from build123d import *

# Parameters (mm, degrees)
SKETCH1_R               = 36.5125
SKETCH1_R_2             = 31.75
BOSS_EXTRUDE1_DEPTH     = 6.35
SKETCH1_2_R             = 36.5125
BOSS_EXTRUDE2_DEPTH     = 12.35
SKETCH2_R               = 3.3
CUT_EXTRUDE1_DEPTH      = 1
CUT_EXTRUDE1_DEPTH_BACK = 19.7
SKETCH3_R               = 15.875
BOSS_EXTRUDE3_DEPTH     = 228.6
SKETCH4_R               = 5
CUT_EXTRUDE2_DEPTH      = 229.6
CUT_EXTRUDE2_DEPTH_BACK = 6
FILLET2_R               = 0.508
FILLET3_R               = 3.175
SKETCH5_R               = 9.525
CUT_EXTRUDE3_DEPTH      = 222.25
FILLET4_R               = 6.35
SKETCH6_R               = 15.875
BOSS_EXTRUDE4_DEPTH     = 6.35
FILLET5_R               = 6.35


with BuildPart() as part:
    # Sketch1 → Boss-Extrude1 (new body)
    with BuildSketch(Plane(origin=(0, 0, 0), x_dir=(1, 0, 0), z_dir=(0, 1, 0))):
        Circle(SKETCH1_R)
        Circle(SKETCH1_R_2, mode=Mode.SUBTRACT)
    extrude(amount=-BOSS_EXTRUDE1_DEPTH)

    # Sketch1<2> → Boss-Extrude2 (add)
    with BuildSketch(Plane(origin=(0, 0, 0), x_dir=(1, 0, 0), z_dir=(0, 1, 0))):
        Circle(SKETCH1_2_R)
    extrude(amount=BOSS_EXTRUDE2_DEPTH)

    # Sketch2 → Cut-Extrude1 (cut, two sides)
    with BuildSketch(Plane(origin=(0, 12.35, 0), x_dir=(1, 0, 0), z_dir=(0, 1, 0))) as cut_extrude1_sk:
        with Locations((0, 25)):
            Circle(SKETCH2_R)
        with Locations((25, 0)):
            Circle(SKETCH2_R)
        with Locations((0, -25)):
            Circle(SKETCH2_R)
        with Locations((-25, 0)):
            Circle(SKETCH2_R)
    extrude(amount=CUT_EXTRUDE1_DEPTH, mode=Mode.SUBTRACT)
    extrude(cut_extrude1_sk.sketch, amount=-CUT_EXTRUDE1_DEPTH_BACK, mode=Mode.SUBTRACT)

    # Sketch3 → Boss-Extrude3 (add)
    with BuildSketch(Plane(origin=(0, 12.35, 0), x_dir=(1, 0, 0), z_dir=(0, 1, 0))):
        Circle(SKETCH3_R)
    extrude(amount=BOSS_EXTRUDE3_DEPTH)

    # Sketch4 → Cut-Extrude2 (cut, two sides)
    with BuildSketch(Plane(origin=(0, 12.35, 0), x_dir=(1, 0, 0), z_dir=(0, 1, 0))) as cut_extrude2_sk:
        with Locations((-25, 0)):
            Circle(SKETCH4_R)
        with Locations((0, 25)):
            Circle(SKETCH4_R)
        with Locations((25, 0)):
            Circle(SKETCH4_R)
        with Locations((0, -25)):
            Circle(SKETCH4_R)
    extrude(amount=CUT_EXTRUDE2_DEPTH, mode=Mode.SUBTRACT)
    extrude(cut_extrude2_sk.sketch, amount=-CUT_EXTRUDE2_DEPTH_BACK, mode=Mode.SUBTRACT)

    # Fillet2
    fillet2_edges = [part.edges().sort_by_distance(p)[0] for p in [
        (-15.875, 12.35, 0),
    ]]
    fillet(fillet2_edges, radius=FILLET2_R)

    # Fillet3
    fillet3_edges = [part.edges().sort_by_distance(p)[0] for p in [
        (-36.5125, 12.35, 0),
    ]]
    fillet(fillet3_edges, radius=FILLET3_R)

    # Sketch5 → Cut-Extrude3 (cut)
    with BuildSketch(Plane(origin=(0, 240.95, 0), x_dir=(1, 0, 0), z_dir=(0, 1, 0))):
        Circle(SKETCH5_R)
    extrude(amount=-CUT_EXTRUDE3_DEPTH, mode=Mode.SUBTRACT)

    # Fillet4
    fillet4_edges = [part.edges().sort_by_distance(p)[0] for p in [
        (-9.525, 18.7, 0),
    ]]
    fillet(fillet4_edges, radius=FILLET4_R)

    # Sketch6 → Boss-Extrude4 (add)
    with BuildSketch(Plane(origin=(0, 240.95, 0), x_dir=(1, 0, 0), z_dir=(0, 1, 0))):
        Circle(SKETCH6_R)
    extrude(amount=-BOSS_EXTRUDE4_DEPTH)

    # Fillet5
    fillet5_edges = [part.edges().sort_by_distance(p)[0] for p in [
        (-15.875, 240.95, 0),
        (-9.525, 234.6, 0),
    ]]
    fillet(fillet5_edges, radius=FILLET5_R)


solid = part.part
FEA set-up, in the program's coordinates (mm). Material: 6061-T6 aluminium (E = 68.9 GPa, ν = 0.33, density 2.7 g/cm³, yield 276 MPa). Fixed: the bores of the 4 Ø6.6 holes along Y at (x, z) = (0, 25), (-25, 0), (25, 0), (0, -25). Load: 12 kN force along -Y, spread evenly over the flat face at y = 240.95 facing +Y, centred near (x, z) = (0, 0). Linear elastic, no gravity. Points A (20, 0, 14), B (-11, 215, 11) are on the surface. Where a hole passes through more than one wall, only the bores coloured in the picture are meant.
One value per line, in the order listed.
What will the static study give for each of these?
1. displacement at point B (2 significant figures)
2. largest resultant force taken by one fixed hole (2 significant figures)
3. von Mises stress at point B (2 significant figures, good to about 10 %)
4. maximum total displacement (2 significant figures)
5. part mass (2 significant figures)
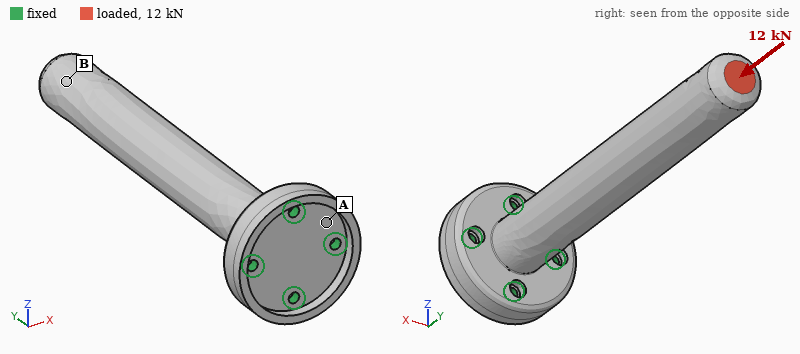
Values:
79 µm
3.3 kN
26 MPa
100 µm
470 g
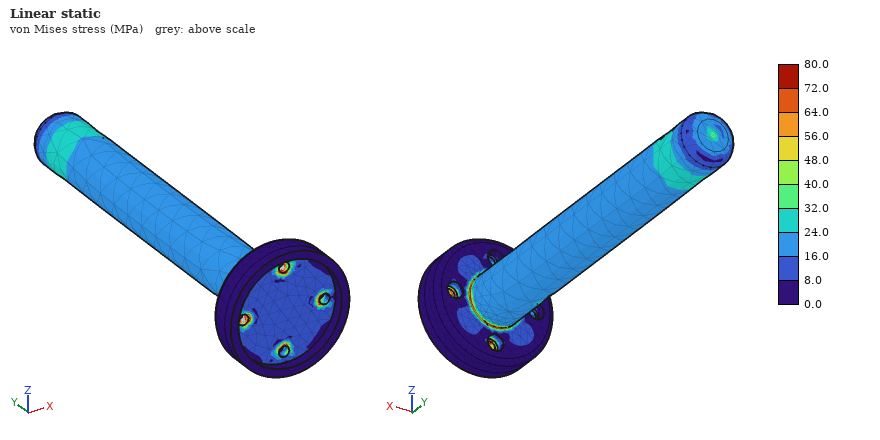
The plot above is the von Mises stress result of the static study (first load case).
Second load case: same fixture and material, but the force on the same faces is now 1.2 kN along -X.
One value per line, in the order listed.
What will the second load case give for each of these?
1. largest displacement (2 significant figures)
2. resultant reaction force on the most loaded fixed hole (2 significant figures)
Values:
1.9 mm
5.9 kN
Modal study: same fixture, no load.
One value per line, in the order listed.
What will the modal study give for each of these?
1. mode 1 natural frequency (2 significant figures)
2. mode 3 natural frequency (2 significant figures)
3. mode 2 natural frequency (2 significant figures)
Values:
440 Hz
2600 Hz
440 Hz
